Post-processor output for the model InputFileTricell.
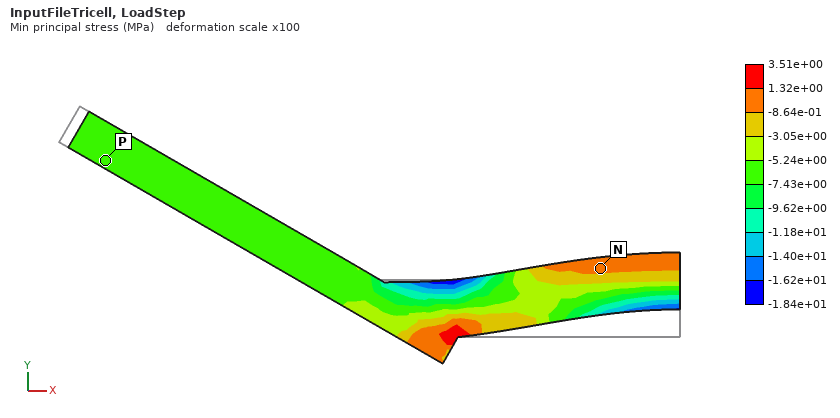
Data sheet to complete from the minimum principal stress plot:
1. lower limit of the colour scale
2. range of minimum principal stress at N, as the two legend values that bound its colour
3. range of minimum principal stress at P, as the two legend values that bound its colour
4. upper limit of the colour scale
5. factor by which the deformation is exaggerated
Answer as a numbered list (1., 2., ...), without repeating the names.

1. -1.84e+01 MPa
2. -8.64e-01 to 1.32e+00 MPa
3. -7.43e+00 to -5.24e+00 MPa
4. 3.51e+00 MPa
5. 100
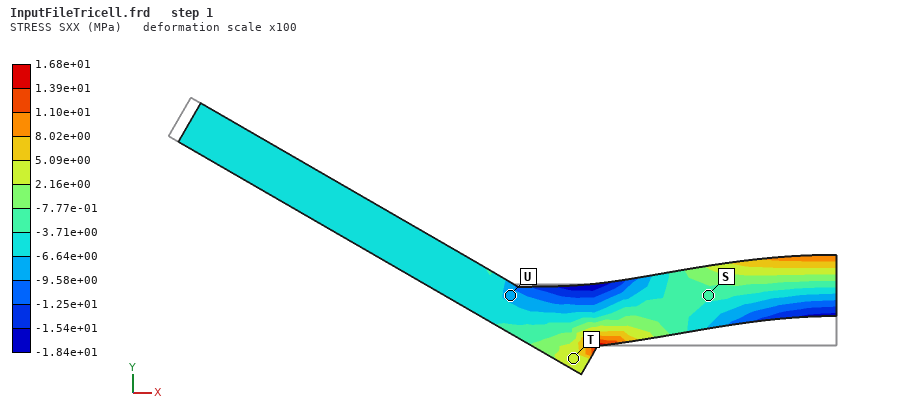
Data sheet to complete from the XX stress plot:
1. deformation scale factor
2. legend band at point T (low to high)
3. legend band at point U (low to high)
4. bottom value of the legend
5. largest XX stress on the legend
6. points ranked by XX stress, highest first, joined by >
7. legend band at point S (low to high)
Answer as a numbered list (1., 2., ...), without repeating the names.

1. 100
2. 2.16e+00 to 5.09e+00 MPa
3. -9.58e+00 to -6.64e+00 MPa
4. -1.84e+01 MPa
5. 1.68e+01 MPa
6. T > S > U
7. -3.71e+00 to -7.77e-01 MPa
